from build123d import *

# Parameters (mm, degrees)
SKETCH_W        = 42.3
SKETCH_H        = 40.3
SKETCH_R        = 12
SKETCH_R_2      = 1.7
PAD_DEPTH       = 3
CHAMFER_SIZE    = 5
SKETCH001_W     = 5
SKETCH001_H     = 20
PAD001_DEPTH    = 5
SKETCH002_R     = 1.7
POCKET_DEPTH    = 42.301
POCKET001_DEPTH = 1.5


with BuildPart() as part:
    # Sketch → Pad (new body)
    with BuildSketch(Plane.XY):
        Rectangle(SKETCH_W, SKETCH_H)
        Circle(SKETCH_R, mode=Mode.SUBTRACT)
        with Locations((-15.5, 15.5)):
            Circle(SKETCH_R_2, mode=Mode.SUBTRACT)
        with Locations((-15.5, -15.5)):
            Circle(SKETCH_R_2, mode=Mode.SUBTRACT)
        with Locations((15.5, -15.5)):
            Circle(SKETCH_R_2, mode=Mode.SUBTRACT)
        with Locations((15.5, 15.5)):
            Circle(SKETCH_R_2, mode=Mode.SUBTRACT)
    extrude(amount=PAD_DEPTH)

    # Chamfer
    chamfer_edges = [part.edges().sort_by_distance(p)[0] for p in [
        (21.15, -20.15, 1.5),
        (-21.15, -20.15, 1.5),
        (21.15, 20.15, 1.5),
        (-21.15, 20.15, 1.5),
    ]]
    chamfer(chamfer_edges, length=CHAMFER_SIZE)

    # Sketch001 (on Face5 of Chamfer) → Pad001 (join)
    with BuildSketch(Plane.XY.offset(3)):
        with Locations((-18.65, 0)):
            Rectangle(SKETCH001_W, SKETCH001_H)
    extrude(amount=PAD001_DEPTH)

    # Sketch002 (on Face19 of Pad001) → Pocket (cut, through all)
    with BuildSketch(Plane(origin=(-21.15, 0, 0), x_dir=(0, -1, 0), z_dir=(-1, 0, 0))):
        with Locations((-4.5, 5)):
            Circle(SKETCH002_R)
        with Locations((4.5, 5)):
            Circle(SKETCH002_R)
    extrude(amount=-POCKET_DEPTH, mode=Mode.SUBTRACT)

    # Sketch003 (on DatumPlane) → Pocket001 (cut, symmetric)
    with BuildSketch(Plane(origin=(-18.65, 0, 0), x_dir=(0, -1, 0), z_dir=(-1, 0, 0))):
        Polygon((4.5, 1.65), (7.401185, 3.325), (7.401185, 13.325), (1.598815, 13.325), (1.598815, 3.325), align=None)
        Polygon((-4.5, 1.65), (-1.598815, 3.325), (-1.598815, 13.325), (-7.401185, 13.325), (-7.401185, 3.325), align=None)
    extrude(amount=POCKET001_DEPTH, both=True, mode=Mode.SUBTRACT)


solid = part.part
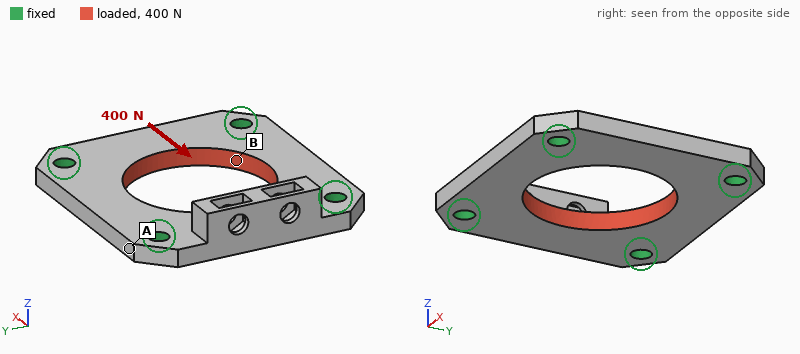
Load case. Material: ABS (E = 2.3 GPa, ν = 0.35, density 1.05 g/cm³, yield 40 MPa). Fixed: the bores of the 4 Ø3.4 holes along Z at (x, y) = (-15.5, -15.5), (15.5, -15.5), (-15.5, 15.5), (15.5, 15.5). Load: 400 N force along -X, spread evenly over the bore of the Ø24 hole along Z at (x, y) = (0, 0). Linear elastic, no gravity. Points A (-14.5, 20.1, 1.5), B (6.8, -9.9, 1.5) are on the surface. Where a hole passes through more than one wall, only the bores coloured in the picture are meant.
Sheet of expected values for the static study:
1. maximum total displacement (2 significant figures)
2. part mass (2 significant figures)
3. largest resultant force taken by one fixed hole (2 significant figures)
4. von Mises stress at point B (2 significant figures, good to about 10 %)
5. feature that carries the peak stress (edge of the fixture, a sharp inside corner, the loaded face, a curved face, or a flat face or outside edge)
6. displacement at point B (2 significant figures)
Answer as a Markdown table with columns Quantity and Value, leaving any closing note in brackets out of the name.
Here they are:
| Quantity | Value |
|---|---|
| maximum total displacement | 41 µm |
| part mass | 4.0 g |
| largest resultant force taken by one fixed hole | 100 N |
| von Mises stress at point B | 4.7 MPa |
| feature that carries the peak stress | edge of the fixture |
| displacement at point B | 20 µm |
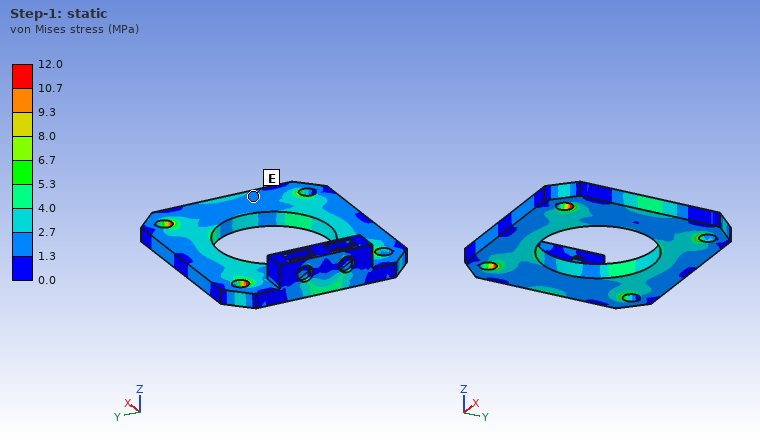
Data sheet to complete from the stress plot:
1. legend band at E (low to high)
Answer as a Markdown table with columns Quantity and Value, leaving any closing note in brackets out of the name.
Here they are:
| Quantity | Value |
|---|---|
| legend band at E | 1.3 to 2.7 MPa |
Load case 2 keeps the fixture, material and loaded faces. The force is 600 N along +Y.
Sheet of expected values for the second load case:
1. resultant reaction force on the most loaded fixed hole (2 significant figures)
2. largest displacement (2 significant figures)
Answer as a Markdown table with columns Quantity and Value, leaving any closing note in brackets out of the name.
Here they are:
| Quantity | Value |
|---|---|
| resultant reaction force on the most loaded fixed hole | 150 N |
| largest displacement | 66 µm |
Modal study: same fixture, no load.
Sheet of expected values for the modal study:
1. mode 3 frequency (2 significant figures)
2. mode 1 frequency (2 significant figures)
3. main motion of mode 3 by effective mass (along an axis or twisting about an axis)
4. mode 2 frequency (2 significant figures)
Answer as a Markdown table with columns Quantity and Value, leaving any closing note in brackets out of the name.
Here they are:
| Quantity | Value |
|---|---|
| mode 3 frequency | 5300 Hz |
| mode 1 frequency | 5000 Hz |
| main motion of mode 3 by effective mass | twisting about X |
| mode 2 frequency | 5100 Hz |
